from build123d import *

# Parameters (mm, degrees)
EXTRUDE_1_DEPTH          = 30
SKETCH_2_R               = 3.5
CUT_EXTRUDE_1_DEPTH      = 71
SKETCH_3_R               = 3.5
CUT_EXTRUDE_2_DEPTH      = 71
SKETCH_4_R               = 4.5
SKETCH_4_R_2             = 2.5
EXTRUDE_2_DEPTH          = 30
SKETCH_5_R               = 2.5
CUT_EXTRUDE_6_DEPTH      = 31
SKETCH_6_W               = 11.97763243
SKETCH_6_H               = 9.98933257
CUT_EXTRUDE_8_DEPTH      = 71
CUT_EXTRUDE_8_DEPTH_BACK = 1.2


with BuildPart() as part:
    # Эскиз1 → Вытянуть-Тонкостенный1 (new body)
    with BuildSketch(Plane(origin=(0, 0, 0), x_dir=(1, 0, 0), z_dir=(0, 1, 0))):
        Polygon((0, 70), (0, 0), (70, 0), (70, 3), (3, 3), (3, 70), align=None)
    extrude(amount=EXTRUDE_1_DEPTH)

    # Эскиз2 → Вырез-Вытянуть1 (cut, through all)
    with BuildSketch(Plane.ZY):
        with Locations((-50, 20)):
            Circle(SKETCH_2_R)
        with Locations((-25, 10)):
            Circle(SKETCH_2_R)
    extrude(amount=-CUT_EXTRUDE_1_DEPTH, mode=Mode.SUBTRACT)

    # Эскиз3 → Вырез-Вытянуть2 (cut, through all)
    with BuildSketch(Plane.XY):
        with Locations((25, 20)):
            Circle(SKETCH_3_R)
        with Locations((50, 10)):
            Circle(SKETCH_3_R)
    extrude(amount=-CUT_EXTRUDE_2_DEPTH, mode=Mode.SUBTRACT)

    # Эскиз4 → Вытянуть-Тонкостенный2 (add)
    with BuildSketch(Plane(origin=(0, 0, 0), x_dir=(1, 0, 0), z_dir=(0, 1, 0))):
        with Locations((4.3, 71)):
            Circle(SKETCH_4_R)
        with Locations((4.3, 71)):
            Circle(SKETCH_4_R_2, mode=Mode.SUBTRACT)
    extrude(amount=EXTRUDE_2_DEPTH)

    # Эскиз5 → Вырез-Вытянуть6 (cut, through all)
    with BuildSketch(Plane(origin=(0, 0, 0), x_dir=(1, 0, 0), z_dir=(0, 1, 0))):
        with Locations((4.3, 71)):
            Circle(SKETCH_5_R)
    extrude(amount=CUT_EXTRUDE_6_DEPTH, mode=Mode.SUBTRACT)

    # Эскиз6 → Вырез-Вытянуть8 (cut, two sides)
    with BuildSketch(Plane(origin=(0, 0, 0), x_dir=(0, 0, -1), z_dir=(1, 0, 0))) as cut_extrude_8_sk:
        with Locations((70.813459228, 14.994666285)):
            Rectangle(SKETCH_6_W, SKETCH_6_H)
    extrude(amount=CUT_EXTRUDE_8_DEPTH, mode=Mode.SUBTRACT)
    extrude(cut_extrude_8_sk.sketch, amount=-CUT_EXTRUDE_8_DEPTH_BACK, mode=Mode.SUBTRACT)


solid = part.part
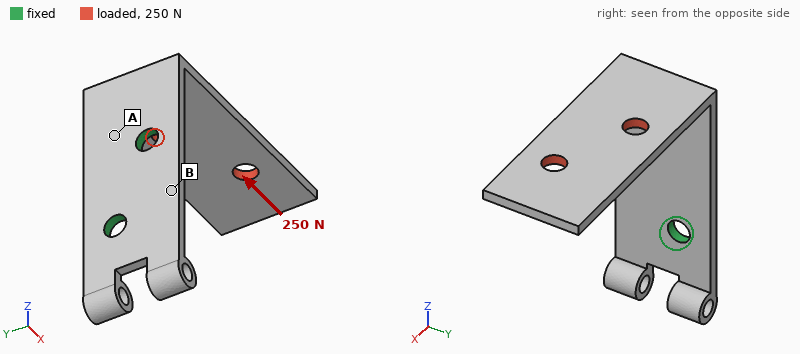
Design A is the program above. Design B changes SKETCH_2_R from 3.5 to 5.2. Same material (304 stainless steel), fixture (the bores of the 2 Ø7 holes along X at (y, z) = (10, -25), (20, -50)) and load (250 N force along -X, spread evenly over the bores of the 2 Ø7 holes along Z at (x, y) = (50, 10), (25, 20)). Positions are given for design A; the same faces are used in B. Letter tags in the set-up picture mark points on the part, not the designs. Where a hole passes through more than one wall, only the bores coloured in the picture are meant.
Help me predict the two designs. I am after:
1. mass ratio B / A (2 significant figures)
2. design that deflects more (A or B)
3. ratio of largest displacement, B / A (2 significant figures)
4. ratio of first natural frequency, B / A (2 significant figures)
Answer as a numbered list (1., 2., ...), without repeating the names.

1. 0.98
2. A
3. 0.83
4. 1.0
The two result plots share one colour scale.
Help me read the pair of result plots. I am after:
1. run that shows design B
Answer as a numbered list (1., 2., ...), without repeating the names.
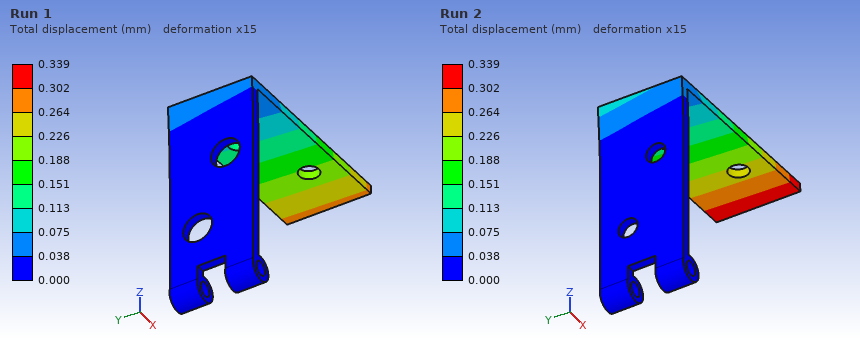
1. Run 1
